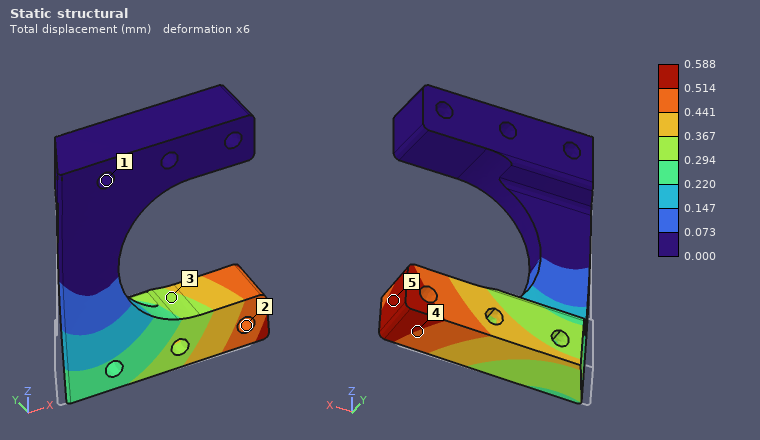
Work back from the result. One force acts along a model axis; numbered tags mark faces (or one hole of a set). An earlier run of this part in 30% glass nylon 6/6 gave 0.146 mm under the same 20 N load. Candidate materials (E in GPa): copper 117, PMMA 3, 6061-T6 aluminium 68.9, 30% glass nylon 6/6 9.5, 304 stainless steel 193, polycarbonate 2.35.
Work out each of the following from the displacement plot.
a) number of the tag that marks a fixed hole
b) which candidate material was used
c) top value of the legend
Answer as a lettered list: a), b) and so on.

a) 1
b) polycarbonate
c) 0.588 mm
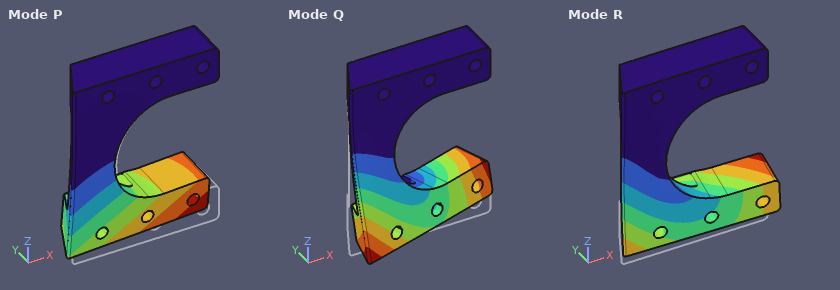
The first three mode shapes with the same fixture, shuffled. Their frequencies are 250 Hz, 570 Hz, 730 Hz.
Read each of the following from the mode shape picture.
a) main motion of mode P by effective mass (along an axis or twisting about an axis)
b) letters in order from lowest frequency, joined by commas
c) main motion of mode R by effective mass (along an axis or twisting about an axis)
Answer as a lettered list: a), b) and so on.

a) along Y
b) P, R, Q
c) along X
